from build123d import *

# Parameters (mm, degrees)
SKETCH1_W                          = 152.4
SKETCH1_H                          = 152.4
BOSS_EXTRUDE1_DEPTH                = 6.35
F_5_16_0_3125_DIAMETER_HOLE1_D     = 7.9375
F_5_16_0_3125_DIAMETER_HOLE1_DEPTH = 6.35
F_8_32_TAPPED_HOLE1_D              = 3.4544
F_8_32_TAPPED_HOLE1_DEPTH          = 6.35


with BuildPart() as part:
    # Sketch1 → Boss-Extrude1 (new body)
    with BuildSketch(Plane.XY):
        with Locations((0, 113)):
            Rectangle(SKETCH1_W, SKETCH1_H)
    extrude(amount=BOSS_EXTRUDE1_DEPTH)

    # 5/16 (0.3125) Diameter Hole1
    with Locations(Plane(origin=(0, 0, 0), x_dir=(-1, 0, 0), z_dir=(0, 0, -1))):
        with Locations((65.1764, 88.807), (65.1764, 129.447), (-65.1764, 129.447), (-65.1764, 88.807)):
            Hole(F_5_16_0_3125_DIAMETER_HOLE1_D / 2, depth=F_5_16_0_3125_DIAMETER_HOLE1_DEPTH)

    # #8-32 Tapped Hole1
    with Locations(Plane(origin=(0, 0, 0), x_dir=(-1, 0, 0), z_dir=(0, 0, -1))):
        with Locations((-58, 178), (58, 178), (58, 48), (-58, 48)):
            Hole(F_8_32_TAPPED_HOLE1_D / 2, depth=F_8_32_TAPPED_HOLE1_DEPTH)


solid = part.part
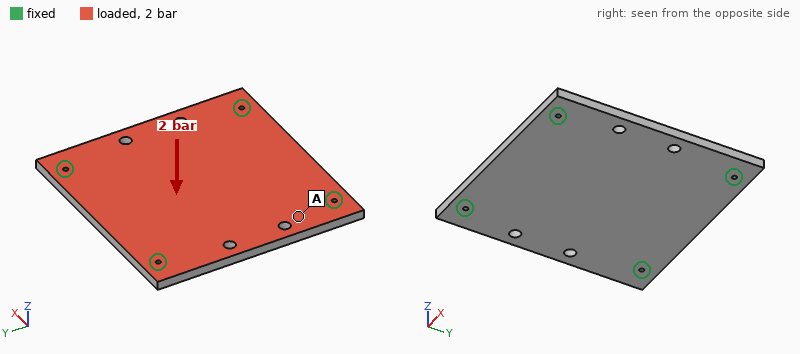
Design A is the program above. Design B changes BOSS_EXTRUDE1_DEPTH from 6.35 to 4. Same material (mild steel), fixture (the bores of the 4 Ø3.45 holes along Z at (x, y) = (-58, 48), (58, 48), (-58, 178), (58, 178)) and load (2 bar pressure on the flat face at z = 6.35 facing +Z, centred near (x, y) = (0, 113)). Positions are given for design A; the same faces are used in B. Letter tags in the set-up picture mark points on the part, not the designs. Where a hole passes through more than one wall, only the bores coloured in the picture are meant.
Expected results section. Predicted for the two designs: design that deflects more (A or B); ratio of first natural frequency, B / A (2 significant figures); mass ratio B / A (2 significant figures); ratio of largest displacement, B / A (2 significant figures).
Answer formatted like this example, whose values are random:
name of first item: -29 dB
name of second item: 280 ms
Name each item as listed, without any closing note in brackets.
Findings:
design that deflects more: B
ratio of first natural frequency, B / A: 0.66
mass ratio B / A: 0.63
ratio of largest displacement, B / A: 3.7
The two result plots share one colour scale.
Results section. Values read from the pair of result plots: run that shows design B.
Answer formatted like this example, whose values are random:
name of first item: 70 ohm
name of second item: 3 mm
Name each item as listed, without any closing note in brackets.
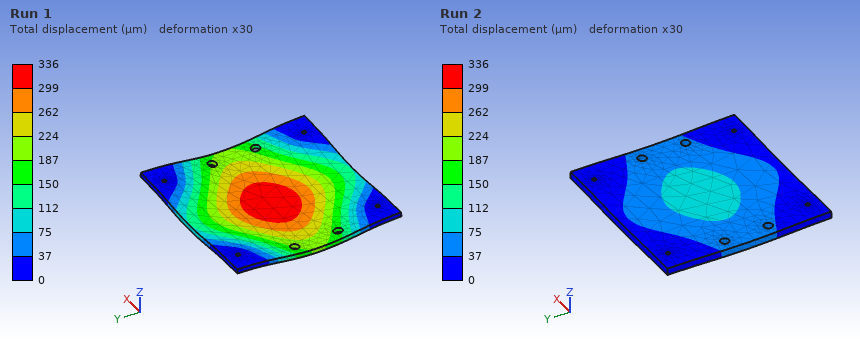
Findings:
run that shows design B: Run 1
